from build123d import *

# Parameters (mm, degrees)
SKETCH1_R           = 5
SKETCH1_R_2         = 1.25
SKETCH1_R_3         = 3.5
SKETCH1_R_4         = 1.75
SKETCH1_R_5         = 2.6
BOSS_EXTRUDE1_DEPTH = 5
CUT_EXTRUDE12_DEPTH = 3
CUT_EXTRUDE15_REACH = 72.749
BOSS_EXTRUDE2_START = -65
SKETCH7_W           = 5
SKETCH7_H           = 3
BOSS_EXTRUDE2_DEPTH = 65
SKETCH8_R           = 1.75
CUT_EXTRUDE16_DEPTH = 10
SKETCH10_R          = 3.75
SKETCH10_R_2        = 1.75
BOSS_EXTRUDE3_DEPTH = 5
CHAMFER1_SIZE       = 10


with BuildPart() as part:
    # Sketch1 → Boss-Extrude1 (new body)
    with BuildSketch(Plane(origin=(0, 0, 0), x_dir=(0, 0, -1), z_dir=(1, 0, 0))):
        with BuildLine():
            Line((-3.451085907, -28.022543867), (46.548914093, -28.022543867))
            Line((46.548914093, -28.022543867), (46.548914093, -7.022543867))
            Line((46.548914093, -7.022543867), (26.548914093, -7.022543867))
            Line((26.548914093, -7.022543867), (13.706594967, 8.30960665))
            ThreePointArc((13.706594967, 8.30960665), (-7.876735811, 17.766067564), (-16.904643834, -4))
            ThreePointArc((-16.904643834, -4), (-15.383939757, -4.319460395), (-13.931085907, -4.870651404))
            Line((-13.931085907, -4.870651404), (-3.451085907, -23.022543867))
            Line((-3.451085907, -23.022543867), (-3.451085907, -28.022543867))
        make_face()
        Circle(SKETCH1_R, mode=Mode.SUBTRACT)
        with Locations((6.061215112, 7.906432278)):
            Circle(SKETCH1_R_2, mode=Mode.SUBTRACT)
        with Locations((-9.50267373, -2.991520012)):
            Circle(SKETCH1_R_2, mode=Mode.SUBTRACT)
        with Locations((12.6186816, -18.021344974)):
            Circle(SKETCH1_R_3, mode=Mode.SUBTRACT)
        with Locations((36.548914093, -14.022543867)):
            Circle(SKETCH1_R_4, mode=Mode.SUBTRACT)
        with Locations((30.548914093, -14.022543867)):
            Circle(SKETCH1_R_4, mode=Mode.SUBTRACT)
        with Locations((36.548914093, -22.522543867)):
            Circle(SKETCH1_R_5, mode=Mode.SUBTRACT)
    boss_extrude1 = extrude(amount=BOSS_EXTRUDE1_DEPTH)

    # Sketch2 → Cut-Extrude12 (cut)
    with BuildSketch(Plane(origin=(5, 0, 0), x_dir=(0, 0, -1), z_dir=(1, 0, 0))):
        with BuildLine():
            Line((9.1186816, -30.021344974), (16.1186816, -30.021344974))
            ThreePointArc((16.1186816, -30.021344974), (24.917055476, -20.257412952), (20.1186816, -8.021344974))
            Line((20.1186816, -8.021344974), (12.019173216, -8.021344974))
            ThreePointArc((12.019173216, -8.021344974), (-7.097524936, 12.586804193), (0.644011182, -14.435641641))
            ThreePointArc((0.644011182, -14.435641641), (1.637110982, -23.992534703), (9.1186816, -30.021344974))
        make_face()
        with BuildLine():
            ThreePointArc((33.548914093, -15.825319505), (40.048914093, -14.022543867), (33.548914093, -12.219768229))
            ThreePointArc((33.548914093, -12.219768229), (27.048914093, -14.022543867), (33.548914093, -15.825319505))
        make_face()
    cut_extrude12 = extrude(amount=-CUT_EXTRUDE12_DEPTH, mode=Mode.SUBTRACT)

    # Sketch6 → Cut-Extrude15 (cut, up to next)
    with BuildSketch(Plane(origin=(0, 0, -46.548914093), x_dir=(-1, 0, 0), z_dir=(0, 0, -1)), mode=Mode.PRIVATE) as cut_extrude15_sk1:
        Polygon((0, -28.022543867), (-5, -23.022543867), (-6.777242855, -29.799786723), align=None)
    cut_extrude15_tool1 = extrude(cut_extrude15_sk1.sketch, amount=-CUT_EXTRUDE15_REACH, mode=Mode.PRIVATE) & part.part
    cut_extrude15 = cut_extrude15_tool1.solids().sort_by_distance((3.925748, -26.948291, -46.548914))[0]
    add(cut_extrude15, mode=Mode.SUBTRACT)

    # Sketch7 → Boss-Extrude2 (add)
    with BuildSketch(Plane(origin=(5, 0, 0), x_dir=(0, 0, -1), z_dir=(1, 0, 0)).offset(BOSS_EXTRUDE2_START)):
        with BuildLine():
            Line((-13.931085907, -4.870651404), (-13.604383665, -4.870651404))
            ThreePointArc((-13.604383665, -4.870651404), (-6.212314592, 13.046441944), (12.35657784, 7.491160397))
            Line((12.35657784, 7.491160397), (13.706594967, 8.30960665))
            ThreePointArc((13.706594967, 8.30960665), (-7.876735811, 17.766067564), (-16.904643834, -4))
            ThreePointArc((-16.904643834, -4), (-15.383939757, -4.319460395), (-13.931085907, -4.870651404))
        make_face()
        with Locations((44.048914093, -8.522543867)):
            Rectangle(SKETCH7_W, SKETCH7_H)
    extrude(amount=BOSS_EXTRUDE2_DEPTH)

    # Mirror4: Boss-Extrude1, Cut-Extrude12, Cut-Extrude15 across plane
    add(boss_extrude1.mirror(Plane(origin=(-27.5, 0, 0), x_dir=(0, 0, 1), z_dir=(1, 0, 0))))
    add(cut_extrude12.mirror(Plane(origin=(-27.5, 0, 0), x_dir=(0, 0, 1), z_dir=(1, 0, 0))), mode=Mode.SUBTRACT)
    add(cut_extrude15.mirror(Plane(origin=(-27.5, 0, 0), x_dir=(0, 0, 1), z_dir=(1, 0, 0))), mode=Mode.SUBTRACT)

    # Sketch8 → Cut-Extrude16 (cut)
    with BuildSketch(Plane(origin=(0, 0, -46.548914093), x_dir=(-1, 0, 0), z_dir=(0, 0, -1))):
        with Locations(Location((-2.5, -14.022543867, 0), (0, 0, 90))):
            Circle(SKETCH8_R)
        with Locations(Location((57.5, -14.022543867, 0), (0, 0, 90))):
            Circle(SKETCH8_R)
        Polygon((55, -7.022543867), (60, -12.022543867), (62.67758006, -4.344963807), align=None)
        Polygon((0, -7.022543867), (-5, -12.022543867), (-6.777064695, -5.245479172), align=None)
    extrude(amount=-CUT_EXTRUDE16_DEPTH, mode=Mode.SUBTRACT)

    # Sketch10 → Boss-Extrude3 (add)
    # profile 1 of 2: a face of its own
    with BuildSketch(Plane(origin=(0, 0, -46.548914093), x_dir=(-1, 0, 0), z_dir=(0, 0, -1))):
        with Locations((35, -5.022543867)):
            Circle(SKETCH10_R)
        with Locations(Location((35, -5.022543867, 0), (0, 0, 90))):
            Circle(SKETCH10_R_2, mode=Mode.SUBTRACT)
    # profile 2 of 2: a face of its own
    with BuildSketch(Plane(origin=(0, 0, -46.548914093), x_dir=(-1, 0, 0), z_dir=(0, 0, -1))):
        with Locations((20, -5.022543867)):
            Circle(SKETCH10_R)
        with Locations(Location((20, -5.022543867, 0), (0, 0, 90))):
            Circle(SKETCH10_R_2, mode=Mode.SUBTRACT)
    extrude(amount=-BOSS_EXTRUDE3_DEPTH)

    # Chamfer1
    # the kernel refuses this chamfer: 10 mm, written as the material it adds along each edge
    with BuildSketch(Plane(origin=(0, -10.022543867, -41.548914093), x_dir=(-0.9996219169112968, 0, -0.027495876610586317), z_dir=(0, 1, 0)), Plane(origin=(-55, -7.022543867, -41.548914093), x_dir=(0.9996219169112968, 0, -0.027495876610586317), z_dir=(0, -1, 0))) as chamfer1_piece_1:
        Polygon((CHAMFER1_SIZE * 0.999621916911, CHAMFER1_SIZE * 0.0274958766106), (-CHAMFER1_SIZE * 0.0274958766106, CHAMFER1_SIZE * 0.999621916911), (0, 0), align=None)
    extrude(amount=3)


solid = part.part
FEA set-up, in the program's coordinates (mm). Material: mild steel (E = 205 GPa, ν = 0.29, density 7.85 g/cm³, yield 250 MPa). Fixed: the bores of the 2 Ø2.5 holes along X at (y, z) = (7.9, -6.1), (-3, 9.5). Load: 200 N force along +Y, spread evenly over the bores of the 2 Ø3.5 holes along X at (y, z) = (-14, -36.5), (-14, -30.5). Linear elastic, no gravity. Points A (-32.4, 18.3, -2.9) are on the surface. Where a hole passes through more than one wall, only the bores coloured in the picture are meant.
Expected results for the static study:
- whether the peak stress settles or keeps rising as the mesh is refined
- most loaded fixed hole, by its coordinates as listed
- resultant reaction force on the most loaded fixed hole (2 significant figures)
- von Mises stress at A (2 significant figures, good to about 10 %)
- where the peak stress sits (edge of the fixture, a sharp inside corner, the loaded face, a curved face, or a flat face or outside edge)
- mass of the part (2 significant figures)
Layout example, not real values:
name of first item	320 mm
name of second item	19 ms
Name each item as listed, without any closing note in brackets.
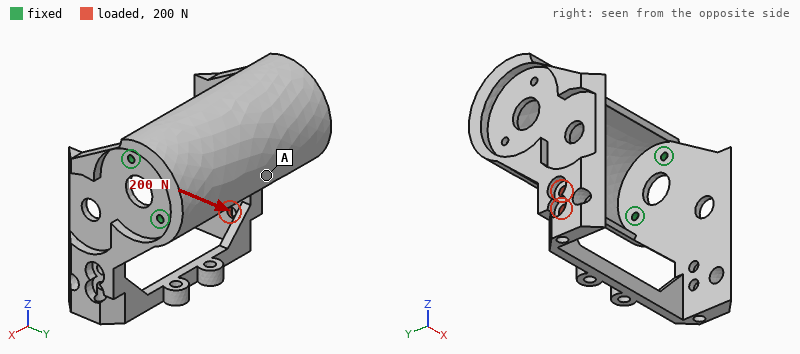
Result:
whether the peak stress settles or keeps rising as the mesh is refined	keeps rising
most loaded fixed hole, by its coordinates as listed	(7.9, -6.1)
resultant reaction force on the most loaded fixed hole	510 N
von Mises stress at A	39 MPa
where the peak stress sits	edge of the fixture
mass of the part	170 g
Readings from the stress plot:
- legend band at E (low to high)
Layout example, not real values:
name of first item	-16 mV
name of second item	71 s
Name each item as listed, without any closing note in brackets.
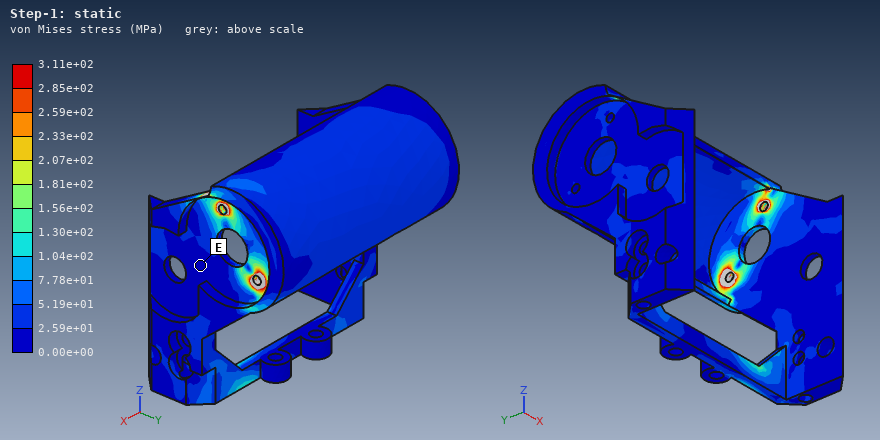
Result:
legend band at E	0.00e+00 to 2.59e+01 MPa
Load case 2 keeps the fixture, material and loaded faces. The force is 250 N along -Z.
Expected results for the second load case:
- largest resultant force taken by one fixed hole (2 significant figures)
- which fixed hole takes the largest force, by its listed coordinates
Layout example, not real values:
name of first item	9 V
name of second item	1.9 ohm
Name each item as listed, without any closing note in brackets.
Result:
largest resultant force taken by one fixed hole	570 N
which fixed hole takes the largest force, by its listed coordinates	(-3, 9.5)
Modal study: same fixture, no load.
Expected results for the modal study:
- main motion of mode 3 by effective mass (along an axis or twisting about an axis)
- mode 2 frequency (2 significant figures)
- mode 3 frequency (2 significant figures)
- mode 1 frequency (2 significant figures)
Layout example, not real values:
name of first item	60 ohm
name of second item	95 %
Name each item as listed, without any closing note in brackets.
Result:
main motion of mode 3 by effective mass	along X
mode 2 frequency	690 Hz
mode 3 frequency	1300 Hz
mode 1 frequency	360 Hz
